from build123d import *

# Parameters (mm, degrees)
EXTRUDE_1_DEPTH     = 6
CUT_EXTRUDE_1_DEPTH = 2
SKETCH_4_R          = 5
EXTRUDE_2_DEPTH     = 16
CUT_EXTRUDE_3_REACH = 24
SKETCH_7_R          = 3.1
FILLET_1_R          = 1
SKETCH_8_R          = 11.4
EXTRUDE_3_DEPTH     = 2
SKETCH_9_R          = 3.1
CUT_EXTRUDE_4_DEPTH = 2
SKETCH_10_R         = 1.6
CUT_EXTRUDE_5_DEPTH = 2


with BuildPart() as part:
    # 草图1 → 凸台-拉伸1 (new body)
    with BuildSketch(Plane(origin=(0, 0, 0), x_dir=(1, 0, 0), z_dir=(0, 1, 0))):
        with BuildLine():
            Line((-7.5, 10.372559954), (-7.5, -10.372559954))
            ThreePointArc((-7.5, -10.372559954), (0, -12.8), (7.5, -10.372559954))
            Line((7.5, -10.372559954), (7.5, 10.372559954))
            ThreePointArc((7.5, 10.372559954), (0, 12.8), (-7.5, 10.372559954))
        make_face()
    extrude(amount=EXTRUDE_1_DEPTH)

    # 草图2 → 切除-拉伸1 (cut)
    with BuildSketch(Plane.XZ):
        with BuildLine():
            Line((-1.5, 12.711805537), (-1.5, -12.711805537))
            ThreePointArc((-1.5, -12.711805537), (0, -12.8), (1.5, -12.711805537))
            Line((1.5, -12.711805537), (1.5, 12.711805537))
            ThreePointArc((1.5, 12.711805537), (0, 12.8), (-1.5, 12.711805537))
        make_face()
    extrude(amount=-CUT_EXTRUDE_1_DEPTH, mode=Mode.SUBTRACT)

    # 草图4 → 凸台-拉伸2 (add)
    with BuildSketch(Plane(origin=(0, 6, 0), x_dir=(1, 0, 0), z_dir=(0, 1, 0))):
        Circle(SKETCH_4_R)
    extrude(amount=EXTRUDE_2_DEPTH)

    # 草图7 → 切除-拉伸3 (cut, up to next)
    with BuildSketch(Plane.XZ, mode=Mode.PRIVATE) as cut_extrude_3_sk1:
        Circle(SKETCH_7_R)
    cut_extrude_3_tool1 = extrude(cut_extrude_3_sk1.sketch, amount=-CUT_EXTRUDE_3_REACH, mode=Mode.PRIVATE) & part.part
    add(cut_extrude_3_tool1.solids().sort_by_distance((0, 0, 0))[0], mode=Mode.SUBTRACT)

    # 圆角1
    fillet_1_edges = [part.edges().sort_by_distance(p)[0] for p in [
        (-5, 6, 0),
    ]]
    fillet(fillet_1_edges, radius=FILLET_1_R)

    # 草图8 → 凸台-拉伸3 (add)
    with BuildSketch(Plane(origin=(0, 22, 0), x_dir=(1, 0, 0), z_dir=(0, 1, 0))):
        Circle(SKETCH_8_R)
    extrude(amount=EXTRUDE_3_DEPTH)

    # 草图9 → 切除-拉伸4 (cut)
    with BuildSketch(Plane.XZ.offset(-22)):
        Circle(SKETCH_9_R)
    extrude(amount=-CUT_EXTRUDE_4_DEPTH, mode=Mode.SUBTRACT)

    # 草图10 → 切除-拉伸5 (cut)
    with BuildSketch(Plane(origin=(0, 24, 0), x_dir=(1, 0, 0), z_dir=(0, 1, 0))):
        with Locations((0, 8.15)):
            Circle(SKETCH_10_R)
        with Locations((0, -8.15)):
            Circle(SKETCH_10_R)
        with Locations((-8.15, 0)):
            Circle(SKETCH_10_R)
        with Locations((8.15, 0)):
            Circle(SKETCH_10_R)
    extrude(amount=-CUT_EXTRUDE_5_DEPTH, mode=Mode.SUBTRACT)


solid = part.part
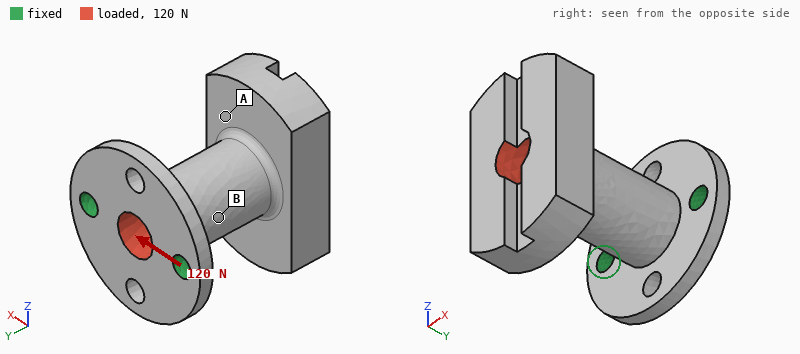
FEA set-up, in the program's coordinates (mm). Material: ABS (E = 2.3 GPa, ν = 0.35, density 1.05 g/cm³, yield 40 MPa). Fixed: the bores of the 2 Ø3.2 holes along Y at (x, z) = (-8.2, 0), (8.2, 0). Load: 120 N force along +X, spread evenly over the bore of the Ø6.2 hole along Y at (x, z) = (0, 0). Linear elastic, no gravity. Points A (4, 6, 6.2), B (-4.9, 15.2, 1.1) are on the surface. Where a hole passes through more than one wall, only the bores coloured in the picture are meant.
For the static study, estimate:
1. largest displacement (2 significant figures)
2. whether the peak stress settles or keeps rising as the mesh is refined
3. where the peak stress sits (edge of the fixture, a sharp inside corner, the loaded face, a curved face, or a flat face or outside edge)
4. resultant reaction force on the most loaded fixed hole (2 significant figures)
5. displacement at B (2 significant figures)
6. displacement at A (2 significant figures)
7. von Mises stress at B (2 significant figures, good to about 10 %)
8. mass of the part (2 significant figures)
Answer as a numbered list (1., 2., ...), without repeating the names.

1. 0.44 mm
2. keeps rising
3. edge of the fixture
4. 120 N
5. 0.15 mm
6. 0.31 mm
7. 5.9 MPa
8. 3.5 g
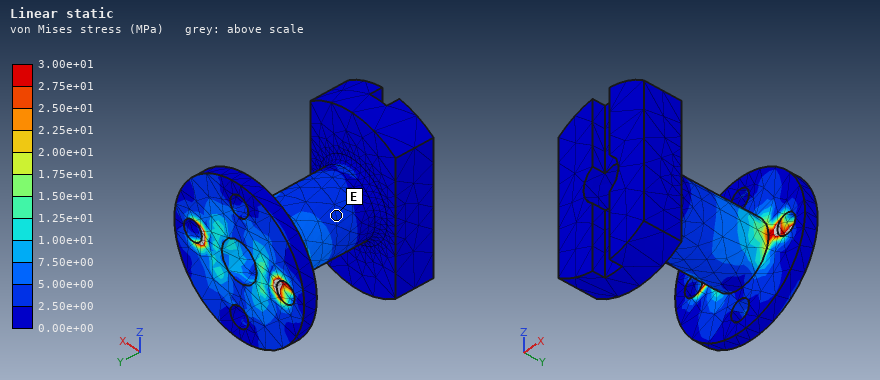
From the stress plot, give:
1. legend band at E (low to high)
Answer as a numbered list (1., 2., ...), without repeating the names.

1. 2.50e+00 to 5.00e+00 MPa
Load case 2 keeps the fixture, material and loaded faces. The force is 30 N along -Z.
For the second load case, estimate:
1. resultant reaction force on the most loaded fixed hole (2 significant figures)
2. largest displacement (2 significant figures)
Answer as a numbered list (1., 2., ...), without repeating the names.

1. 15 N
2. 0.48 mm
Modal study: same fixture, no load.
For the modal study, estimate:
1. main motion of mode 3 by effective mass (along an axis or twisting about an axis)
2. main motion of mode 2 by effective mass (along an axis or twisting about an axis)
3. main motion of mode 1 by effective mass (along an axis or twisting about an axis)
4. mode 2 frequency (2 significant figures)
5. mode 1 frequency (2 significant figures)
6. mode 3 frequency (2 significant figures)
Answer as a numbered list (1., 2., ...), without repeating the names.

1. twisting about Y
2. along X
3. along Z
4. 1300 Hz
5. 670 Hz
6. 2600 Hz
